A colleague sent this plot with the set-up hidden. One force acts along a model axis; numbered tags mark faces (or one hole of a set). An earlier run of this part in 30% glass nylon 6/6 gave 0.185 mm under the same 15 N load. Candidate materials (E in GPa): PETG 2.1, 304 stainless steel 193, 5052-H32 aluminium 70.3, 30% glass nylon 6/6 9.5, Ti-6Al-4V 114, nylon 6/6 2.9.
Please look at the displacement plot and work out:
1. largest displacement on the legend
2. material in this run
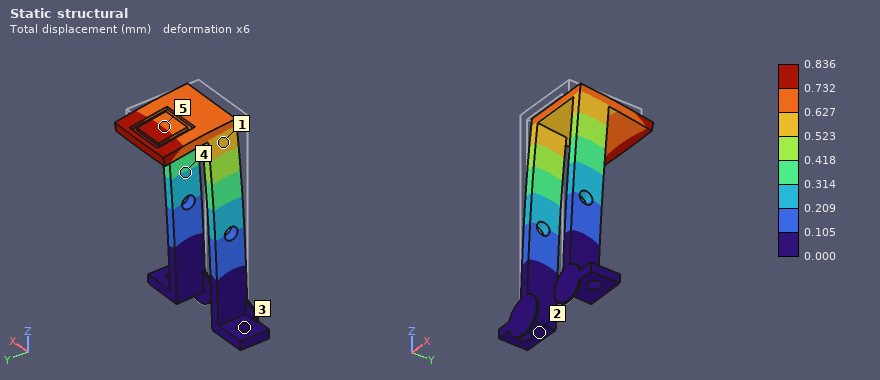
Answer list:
0.836 mm
PETG
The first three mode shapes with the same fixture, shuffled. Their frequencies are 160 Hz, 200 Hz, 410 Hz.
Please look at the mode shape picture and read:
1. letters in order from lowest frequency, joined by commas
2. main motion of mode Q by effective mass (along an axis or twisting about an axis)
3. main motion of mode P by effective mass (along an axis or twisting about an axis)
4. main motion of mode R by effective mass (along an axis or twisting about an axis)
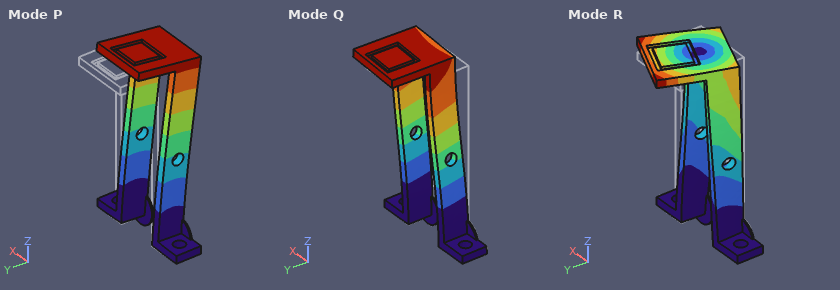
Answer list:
Q, P, R
along X
along Y
twisting about Z
